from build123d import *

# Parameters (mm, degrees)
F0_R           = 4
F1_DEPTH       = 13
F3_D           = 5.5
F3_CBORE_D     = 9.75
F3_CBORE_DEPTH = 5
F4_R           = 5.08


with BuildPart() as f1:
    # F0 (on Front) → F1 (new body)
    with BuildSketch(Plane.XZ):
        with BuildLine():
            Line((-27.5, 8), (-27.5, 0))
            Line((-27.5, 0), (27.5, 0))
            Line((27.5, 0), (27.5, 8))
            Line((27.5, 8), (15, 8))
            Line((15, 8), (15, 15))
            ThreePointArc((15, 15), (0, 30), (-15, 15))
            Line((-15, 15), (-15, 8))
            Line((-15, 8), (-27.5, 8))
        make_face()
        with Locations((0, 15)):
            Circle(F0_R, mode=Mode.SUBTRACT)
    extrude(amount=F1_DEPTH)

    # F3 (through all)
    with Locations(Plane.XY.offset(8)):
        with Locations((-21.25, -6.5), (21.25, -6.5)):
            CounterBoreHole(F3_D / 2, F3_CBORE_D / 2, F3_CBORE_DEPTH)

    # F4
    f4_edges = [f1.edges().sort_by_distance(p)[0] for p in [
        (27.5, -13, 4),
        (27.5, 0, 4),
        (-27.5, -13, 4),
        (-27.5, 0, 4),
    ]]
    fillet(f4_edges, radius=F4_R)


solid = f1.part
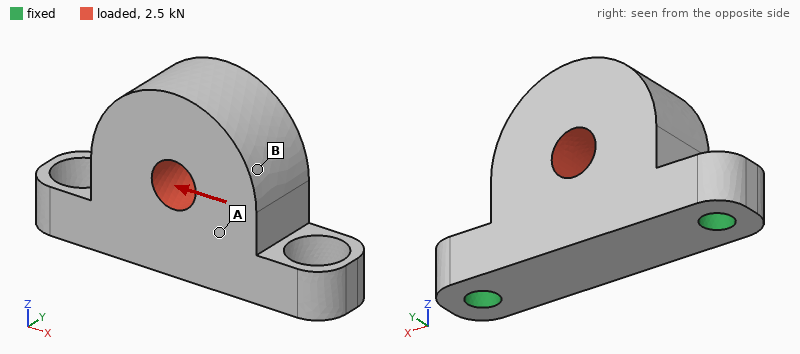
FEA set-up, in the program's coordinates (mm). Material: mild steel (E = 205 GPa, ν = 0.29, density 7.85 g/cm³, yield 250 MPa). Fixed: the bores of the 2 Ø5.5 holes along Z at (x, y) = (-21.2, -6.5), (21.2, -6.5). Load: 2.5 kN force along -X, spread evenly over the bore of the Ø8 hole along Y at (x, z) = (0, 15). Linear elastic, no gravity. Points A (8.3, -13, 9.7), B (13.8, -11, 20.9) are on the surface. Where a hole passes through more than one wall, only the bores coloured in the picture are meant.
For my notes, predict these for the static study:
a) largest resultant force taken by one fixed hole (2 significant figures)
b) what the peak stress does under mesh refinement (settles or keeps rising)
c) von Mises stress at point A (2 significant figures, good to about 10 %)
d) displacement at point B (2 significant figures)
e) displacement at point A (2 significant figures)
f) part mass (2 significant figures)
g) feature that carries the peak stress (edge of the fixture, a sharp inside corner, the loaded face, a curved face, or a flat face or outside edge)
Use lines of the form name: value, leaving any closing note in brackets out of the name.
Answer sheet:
largest resultant force taken by one fixed hole: 1.5 kN
what the peak stress does under mesh refinement: keeps rising
von Mises stress at point A: 13 MPa
displacement at point B: 4.2 µm
displacement at point A: 2.0 µm
part mass: 89 g
feature that carries the peak stress: edge of the fixture
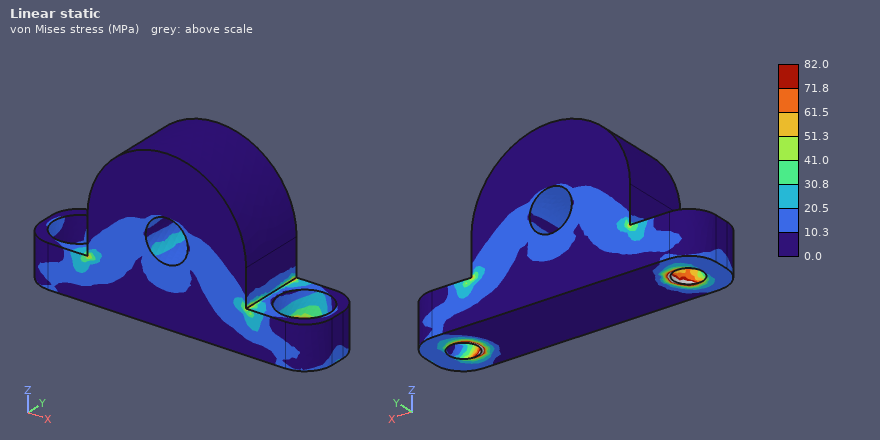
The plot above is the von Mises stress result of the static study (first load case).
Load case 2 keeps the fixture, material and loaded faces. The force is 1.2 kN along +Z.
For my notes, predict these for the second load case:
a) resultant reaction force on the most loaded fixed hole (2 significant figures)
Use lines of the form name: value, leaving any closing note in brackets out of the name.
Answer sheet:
resultant reaction force on the most loaded fixed hole: 730 N
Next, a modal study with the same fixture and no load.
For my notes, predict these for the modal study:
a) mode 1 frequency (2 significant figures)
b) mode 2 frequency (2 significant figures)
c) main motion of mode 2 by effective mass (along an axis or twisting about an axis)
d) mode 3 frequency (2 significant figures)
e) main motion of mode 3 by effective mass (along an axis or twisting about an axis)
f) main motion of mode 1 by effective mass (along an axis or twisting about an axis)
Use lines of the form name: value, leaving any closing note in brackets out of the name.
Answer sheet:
mode 1 frequency: 4000 Hz
mode 2 frequency: 14 kHz
main motion of mode 2 by effective mass: along Z
mode 3 frequency: 15 kHz
main motion of mode 3 by effective mass: along X
main motion of mode 1 by effective mass: along Y
